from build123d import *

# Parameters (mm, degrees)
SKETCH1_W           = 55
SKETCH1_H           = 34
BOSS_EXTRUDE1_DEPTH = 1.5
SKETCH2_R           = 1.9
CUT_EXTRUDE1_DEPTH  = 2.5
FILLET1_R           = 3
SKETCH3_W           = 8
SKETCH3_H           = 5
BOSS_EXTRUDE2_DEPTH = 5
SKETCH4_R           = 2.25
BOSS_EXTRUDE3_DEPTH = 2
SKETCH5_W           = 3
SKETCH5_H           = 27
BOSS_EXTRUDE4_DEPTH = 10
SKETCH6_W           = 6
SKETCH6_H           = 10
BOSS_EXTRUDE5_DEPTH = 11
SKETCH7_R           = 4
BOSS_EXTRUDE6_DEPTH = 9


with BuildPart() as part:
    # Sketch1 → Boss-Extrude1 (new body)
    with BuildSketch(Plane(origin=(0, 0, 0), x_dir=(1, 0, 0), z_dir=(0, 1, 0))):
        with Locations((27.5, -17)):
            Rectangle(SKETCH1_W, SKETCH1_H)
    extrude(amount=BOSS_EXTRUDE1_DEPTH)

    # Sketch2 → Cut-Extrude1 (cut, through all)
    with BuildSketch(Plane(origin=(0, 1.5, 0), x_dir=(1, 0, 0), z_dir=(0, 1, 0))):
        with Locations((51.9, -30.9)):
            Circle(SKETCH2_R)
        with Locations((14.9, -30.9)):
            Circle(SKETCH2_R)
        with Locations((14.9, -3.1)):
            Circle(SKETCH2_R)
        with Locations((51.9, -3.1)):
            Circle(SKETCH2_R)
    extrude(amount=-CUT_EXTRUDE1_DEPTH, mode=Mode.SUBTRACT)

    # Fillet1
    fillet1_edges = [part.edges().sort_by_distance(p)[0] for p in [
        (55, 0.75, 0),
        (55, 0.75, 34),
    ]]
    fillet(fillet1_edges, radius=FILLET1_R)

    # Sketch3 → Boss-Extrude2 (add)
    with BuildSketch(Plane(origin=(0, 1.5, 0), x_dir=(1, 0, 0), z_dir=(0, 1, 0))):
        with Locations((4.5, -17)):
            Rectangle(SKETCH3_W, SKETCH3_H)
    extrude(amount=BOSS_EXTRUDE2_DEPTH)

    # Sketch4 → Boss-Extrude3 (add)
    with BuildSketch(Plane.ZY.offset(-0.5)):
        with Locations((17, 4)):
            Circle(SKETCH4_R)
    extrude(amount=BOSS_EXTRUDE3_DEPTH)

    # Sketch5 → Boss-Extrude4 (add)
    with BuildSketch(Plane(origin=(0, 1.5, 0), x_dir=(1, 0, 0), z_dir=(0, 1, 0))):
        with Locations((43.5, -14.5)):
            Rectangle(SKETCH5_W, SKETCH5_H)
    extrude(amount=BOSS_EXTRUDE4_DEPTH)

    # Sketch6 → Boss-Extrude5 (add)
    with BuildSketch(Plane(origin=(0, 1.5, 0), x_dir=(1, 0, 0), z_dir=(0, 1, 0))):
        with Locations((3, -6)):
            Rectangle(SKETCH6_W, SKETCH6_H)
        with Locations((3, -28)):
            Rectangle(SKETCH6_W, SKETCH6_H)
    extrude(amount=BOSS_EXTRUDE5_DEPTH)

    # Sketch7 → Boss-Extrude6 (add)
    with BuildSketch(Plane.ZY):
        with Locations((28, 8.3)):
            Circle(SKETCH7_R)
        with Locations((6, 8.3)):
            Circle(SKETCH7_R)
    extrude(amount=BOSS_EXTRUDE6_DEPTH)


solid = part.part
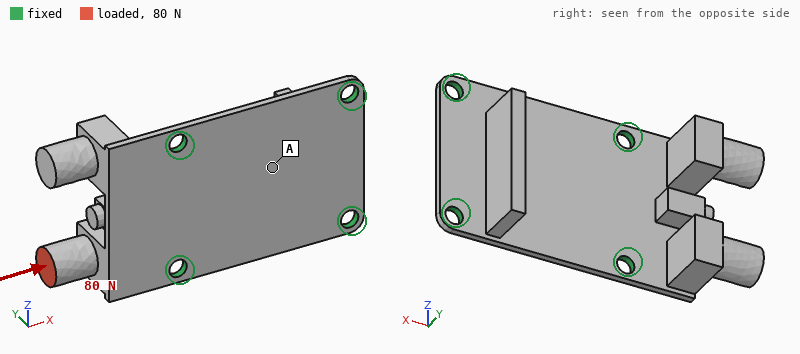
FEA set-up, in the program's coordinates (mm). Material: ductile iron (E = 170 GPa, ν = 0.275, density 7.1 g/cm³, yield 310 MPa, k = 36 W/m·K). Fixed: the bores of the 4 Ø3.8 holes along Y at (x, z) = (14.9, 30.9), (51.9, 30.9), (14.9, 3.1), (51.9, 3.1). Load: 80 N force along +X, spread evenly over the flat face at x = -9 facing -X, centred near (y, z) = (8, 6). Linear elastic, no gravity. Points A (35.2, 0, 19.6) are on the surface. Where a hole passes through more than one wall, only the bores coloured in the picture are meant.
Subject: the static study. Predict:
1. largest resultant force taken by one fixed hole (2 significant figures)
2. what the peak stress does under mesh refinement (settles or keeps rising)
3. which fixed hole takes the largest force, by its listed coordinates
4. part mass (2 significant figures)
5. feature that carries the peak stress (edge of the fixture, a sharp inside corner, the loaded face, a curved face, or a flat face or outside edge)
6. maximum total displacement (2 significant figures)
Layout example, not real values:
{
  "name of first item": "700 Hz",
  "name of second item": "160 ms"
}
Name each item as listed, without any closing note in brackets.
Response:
{
  "largest resultant force taken by one fixed hole": "65 N",
  "what the peak stress does under mesh refinement": "keeps rising",
  "which fixed hole takes the largest force, by its listed coordinates": "(14.9, 3.1)",
  "part mass": "43 g",
  "feature that carries the peak stress": "edge of the fixture",
  "maximum total displacement": "96 µm"
}
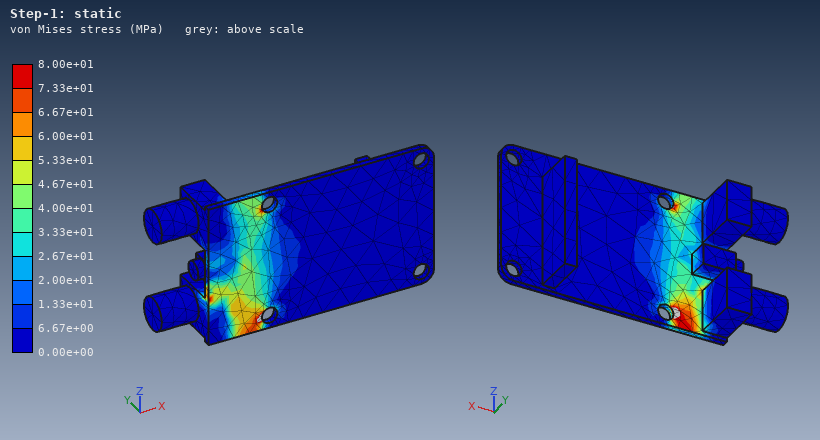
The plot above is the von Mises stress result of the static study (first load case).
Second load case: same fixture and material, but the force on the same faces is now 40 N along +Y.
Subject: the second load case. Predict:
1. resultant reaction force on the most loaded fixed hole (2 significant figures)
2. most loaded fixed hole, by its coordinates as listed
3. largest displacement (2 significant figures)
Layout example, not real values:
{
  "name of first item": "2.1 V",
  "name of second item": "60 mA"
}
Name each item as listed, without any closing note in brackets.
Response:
{
  "resultant reaction force on the most loaded fixed hole": "37 N",
  "most loaded fixed hole, by its coordinates as listed": "(14.9, 3.1)",
  "largest displacement": "0.12 mm"
}
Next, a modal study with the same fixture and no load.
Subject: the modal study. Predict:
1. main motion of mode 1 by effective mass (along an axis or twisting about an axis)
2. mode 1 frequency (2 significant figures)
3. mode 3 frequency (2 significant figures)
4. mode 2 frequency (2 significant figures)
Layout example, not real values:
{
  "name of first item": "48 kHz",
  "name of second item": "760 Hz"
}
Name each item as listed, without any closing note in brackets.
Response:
{
  "main motion of mode 1 by effective mass": "along Y",
  "mode 1 frequency": "1200 Hz",
  "mode 3 frequency": "3500 Hz",
  "mode 2 frequency": "2400 Hz"
}
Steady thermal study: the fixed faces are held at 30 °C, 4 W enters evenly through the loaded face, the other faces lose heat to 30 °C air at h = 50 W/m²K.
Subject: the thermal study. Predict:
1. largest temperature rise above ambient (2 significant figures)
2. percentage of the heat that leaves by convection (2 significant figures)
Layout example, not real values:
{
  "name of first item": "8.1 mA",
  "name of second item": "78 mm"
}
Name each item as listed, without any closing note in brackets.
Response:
{
  "largest temperature rise above ambient": "56 K",
  "percentage of the heat that leaves by convection": "49 %"
}
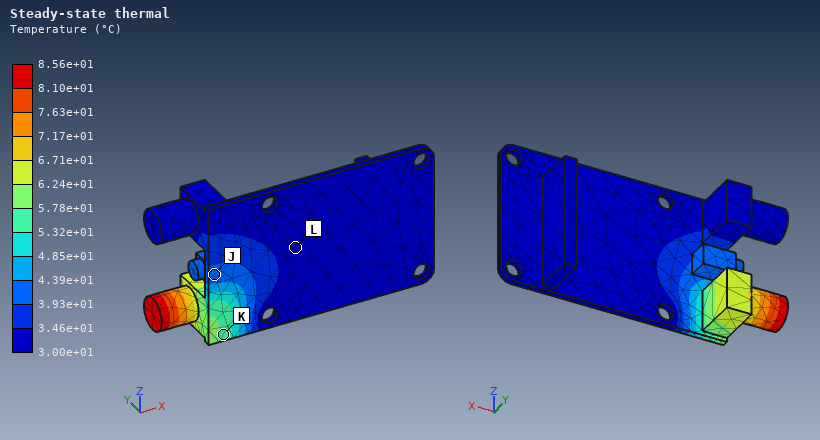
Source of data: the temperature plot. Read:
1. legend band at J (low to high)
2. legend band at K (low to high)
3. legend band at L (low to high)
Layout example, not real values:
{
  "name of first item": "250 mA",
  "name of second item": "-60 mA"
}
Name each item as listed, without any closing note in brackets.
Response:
{
  "legend band at J": "3.93e+01 to 4.39e+01 °C",
  "legend band at K": "5.32e+01 to 5.78e+01 °C",
  "legend band at L": "3.00e+01 to 3.46e+01 °C"
}
